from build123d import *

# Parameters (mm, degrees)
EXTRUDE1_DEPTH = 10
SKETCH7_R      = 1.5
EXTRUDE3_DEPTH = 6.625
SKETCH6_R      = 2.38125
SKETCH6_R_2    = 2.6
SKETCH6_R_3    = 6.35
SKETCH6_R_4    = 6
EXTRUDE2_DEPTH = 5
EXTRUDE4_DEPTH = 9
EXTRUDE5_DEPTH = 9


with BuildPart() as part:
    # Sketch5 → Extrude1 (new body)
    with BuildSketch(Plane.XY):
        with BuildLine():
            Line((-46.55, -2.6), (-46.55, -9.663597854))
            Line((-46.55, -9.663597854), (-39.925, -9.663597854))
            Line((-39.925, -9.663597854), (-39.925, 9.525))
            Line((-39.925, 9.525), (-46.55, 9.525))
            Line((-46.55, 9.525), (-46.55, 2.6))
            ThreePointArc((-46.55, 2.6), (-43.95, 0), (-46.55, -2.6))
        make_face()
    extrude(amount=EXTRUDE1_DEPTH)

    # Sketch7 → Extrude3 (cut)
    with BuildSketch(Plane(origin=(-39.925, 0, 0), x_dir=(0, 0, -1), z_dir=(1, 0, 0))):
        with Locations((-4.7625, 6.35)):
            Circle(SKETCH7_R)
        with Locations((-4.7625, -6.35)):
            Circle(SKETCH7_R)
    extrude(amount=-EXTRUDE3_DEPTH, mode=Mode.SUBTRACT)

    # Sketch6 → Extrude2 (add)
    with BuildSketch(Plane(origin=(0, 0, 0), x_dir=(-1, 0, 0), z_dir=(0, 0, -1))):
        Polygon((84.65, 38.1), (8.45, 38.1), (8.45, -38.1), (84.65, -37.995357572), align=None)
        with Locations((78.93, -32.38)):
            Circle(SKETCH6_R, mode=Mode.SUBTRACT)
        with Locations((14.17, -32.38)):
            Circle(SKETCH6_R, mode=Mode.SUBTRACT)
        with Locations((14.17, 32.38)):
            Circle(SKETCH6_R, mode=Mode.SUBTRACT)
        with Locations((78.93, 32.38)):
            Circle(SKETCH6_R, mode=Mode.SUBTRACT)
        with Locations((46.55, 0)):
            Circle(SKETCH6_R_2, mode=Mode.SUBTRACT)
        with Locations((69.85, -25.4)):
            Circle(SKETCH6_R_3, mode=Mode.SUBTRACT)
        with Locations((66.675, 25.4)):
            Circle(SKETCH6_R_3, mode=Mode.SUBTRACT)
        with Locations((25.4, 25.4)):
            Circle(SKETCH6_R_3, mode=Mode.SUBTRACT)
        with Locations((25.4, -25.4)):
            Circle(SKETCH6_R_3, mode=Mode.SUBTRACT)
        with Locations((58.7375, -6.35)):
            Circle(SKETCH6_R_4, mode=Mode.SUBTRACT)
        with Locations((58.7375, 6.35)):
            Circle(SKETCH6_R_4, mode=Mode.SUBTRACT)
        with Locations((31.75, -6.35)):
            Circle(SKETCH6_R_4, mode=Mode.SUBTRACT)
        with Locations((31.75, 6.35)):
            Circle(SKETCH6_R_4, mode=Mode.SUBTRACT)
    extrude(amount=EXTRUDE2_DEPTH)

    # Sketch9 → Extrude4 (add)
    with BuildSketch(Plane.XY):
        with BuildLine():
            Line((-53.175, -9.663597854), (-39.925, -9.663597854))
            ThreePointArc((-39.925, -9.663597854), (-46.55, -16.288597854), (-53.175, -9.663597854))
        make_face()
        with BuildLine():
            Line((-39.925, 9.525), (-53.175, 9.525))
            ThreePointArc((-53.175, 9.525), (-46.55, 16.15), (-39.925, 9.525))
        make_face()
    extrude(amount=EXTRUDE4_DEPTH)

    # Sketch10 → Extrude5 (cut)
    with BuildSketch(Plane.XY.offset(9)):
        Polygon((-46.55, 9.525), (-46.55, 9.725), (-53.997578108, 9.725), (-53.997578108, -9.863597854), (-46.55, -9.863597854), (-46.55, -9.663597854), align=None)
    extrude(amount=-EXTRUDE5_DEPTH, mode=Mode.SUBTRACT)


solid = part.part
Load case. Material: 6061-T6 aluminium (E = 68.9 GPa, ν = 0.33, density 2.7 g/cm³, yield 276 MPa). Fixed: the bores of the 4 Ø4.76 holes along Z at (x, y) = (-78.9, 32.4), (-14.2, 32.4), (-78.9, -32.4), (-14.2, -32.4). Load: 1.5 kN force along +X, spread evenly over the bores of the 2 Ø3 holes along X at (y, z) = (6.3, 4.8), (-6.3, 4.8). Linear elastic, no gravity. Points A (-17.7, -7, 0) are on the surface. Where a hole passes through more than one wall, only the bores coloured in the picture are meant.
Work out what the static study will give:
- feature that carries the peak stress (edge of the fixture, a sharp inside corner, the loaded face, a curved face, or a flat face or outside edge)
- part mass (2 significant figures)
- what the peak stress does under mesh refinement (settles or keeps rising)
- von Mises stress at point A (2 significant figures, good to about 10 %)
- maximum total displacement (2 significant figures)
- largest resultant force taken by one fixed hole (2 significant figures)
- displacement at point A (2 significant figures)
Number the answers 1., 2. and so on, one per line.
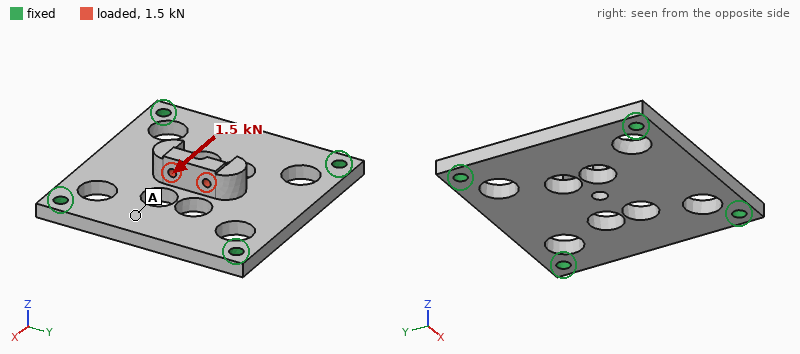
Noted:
1. a sharp inside corner
2. 70 g
3. keeps rising
4. 7.4 MPa
5. 42 µm
6. 440 N
7. 14 µm
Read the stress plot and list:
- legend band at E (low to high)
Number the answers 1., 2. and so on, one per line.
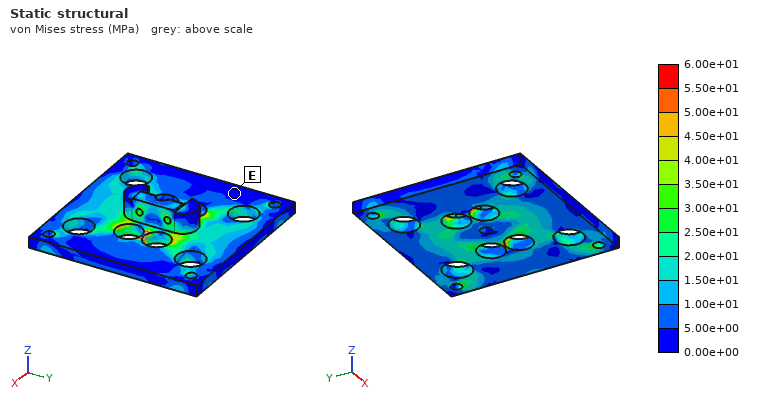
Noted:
1. 0.00e+00 to 5.00e+00 MPa
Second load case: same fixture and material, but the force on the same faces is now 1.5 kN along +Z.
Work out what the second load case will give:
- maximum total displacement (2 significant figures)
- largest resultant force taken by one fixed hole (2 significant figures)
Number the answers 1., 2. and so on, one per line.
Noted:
1. 0.12 mm
2. 430 N
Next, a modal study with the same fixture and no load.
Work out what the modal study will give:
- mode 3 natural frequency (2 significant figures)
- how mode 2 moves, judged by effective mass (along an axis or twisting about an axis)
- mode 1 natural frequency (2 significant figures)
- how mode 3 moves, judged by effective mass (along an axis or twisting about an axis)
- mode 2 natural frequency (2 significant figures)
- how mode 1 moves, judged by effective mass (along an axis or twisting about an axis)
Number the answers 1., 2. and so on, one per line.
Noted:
1. 6300 Hz
2. twisting about X
3. 3500 Hz
4. twisting about Y
5. 5900 Hz
6. along Z
